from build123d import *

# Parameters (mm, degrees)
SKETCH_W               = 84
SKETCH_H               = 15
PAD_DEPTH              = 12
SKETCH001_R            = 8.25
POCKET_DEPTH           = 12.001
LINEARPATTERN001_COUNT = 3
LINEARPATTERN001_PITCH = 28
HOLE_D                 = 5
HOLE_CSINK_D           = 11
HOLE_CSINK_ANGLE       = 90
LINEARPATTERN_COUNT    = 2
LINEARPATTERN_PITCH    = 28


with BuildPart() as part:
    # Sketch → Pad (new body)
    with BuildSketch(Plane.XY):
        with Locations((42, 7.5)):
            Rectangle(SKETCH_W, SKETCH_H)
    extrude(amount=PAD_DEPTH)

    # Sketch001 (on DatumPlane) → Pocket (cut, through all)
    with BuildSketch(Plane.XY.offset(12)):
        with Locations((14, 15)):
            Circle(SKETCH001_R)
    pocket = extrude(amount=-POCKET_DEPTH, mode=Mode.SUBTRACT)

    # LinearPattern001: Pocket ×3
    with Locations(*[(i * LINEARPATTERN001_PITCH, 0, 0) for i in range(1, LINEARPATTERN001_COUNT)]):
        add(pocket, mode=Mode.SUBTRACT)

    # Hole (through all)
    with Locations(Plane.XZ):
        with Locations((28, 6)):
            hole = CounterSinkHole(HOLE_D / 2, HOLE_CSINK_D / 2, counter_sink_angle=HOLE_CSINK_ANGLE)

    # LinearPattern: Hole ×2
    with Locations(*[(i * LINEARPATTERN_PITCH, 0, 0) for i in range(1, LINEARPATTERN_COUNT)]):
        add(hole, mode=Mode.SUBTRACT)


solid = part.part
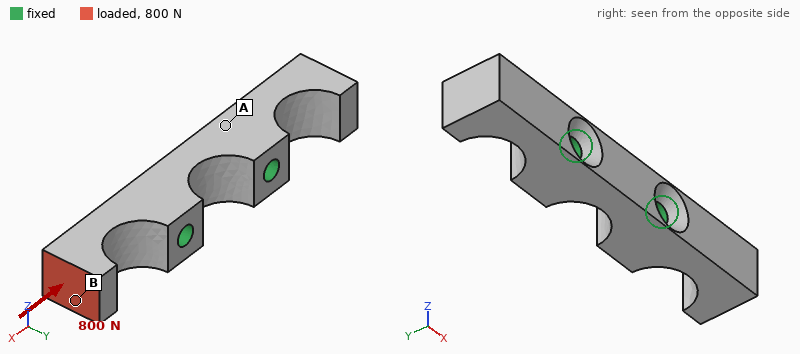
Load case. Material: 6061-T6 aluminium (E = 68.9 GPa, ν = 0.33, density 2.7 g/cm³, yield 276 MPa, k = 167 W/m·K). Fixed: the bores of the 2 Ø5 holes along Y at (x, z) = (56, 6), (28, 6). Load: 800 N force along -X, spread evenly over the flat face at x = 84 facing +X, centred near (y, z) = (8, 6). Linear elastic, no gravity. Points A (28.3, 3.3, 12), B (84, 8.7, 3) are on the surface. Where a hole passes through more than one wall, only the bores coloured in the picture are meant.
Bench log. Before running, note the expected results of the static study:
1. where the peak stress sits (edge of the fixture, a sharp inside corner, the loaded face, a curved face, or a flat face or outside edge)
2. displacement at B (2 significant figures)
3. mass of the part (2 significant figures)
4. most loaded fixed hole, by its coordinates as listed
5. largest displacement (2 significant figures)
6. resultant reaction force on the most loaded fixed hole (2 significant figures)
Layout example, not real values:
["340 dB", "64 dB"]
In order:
["a curved face", "28 µm", "28 g", "(56, 6)", "35 µm", "780 N"]
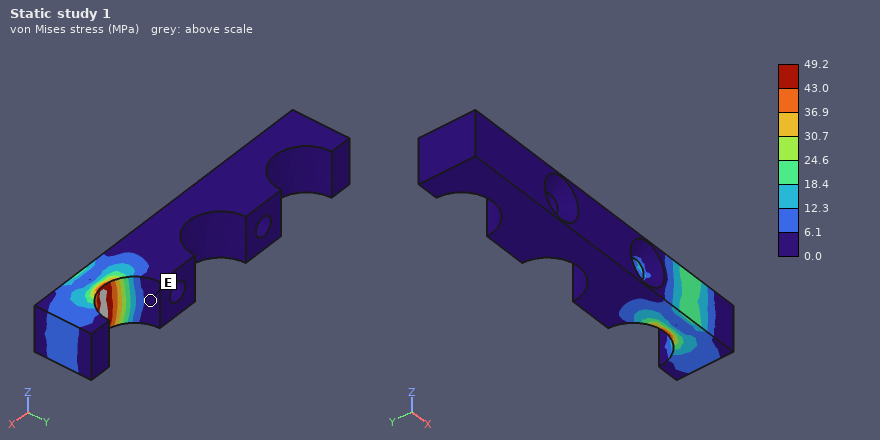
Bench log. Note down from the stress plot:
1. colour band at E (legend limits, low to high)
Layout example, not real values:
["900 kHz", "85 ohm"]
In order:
["0.0 to 6.1 MPa"]
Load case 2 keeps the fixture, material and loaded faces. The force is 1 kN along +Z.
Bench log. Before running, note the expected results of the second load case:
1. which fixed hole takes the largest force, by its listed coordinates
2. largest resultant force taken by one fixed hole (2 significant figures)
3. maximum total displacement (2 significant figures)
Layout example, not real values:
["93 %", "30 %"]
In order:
["(56, 6)", "1.3 kN", "0.15 mm"]
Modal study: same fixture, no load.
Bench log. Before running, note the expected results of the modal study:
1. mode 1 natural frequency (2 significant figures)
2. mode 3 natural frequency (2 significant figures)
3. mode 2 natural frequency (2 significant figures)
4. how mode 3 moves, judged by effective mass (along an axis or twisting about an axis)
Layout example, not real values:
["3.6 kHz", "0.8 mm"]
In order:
["7200 Hz", "8200 Hz", "7200 Hz", "along Z"]
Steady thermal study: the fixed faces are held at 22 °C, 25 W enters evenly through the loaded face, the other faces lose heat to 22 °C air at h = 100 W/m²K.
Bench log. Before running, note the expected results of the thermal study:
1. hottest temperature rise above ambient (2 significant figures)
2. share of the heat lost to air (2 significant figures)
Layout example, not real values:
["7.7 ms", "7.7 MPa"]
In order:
["38 K", "10 %"]
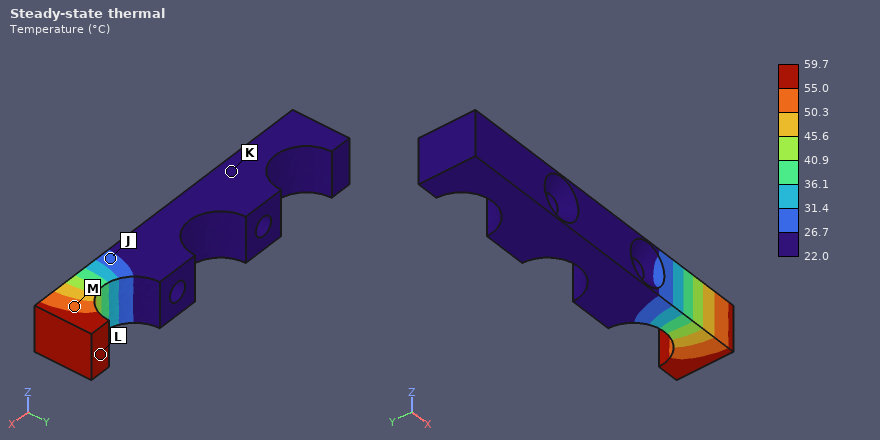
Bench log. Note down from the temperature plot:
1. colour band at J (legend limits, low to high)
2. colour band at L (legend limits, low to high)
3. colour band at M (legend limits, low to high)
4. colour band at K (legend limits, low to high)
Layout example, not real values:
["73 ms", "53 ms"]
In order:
["26.7 to 31.4 °C", "55.0 to 59.7 °C", "50.3 to 55.0 °C", "22.0 to 26.7 °C"]
